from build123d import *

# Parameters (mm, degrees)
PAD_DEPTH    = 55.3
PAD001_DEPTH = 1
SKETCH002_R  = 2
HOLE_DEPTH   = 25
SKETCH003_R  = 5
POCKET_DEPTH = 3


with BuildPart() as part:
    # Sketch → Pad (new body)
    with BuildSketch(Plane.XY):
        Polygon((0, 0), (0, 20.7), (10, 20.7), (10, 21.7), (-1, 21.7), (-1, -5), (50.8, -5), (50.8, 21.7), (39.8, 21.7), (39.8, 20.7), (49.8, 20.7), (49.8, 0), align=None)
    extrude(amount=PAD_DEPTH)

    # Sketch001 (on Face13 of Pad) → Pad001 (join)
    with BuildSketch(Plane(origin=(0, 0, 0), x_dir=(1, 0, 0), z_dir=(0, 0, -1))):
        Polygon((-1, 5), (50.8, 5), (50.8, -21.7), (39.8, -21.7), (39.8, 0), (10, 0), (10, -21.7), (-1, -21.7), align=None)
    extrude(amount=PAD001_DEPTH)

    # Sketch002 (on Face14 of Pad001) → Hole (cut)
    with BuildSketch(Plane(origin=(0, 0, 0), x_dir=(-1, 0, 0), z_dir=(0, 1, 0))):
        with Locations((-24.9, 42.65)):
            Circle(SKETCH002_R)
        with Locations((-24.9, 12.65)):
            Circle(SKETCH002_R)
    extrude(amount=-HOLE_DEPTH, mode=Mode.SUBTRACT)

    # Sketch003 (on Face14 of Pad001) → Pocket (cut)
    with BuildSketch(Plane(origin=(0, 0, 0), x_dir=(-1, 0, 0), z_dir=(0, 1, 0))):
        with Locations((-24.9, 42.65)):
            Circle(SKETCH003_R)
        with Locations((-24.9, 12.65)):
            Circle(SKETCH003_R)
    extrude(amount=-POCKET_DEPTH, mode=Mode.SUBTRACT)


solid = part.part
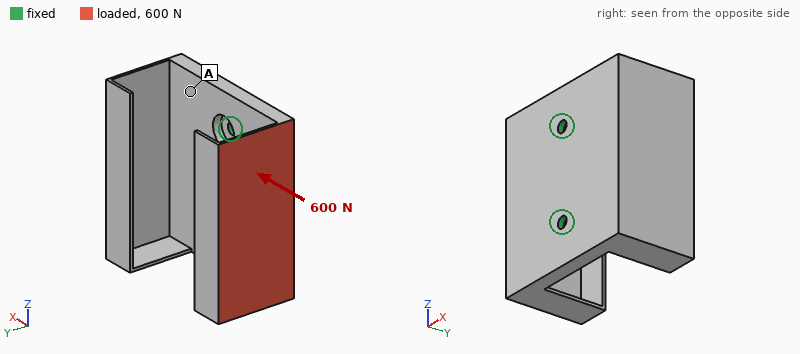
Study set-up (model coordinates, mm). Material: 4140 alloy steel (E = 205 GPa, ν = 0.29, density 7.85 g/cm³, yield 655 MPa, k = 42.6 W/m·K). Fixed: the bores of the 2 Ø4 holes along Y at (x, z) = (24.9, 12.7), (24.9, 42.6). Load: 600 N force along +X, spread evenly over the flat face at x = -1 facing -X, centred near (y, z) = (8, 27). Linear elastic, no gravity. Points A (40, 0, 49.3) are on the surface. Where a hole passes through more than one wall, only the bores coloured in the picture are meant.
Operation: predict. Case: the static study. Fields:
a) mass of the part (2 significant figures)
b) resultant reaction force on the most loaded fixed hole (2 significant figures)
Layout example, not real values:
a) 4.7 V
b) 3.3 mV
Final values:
a) 140 g
b) 320 N
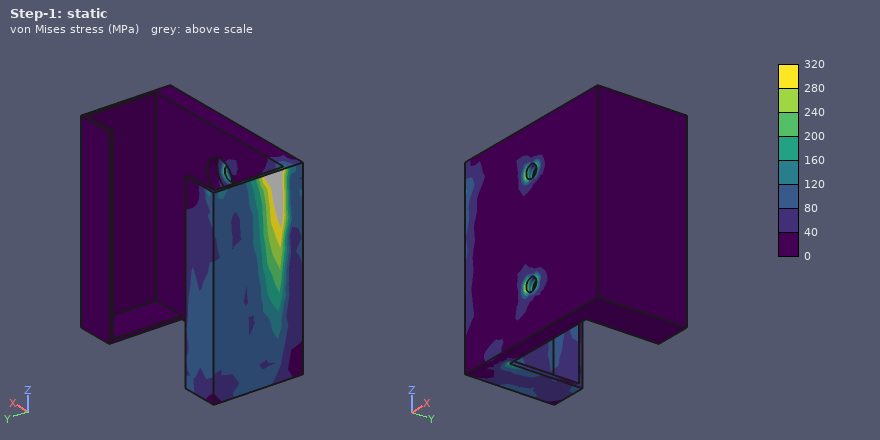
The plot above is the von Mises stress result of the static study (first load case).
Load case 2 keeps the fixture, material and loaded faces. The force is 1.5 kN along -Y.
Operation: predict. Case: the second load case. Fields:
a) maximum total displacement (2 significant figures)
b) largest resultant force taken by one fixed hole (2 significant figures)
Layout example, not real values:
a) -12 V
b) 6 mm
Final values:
a) 0.45 mm
b) 790 N
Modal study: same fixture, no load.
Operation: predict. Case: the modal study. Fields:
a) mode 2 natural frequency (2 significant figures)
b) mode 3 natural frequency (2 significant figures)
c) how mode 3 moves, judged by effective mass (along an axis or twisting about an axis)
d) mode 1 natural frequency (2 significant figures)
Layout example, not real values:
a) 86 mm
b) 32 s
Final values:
a) 1300 Hz
b) 1700 Hz
c) twisting about Z
d) 1200 Hz
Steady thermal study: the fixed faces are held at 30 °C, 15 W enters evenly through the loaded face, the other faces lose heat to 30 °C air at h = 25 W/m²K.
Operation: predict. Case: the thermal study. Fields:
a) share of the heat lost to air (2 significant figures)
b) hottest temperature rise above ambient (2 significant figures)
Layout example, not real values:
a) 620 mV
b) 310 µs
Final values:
a) 42 %
b) 63 K
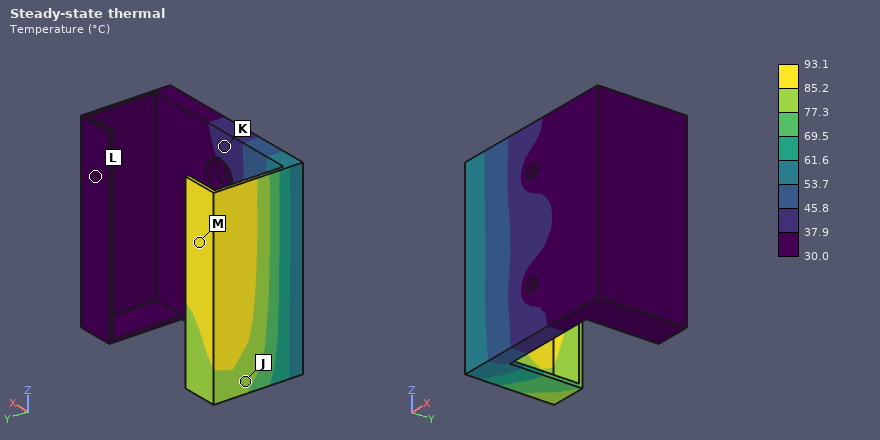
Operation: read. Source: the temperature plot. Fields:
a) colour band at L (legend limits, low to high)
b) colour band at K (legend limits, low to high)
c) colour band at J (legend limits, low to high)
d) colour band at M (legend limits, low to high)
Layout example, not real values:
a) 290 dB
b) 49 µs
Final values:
a) 30.0 to 37.9 °C
b) 37.9 to 45.8 °C
c) 77.3 to 85.2 °C
d) 85.2 to 93.1 °C
